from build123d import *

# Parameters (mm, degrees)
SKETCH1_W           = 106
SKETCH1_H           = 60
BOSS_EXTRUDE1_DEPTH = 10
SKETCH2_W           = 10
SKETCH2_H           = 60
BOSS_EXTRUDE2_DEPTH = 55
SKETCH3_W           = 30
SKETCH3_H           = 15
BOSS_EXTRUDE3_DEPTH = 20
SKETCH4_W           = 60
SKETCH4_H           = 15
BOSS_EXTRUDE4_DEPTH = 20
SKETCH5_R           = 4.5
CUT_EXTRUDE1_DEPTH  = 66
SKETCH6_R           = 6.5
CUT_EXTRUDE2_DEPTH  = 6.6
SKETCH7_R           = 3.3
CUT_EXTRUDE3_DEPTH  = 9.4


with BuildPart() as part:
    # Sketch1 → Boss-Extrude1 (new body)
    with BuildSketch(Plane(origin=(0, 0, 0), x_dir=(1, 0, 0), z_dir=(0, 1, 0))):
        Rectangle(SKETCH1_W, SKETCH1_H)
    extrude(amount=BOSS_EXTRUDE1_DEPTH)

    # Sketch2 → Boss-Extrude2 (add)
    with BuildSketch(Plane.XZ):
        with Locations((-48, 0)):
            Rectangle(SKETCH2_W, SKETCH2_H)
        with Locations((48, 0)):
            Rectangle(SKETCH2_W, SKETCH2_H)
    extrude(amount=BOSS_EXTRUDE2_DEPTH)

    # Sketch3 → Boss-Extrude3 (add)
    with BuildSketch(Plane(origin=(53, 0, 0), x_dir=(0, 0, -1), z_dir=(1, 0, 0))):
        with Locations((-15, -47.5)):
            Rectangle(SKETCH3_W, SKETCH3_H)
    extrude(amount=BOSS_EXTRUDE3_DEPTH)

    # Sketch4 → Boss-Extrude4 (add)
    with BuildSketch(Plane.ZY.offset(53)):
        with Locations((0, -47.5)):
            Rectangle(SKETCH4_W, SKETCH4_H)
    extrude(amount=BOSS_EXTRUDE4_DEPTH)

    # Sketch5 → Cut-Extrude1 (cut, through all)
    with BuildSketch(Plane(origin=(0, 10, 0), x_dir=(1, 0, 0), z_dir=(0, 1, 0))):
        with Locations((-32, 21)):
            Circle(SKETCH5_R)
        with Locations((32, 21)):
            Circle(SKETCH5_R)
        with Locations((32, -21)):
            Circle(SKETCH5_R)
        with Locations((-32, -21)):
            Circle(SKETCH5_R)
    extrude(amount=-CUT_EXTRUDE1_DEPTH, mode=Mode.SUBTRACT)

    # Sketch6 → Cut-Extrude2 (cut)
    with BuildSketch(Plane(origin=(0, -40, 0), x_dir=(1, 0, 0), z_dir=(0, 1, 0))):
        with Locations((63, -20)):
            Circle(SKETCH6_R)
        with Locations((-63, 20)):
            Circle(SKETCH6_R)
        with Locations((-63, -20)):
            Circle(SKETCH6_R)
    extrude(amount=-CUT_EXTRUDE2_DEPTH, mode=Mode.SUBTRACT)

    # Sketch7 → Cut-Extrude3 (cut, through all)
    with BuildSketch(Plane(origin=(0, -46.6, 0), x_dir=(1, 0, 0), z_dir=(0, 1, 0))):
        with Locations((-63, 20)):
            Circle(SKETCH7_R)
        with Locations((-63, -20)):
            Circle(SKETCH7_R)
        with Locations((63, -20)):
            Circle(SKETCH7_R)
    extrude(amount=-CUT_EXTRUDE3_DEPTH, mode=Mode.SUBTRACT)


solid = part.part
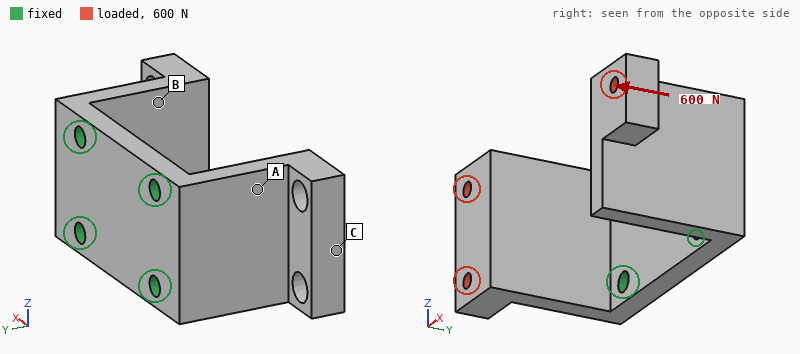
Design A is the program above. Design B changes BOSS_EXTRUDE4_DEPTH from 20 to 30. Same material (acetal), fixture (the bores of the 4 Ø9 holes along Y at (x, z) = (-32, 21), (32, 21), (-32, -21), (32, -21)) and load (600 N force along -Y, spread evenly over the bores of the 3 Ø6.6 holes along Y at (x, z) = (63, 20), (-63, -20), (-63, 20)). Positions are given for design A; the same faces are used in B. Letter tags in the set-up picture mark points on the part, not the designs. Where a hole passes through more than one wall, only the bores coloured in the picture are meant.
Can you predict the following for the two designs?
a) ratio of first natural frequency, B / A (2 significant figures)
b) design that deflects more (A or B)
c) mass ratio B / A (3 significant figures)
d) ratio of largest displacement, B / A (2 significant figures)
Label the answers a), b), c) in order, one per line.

a) 0.83
b) B
c) 1.06
d) 1.1
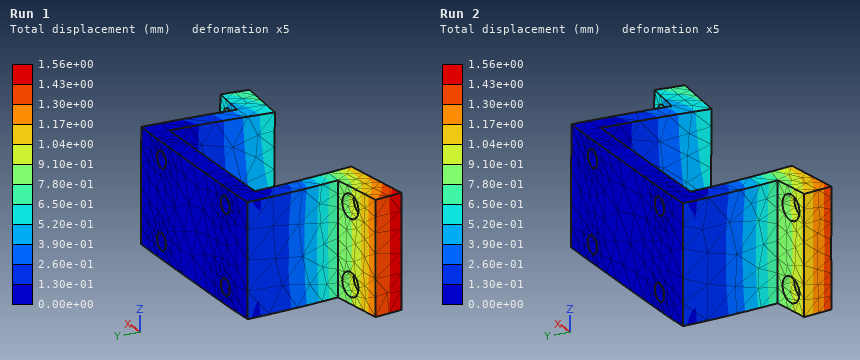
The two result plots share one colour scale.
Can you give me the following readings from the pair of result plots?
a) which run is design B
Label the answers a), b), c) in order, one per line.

a) Run 1
